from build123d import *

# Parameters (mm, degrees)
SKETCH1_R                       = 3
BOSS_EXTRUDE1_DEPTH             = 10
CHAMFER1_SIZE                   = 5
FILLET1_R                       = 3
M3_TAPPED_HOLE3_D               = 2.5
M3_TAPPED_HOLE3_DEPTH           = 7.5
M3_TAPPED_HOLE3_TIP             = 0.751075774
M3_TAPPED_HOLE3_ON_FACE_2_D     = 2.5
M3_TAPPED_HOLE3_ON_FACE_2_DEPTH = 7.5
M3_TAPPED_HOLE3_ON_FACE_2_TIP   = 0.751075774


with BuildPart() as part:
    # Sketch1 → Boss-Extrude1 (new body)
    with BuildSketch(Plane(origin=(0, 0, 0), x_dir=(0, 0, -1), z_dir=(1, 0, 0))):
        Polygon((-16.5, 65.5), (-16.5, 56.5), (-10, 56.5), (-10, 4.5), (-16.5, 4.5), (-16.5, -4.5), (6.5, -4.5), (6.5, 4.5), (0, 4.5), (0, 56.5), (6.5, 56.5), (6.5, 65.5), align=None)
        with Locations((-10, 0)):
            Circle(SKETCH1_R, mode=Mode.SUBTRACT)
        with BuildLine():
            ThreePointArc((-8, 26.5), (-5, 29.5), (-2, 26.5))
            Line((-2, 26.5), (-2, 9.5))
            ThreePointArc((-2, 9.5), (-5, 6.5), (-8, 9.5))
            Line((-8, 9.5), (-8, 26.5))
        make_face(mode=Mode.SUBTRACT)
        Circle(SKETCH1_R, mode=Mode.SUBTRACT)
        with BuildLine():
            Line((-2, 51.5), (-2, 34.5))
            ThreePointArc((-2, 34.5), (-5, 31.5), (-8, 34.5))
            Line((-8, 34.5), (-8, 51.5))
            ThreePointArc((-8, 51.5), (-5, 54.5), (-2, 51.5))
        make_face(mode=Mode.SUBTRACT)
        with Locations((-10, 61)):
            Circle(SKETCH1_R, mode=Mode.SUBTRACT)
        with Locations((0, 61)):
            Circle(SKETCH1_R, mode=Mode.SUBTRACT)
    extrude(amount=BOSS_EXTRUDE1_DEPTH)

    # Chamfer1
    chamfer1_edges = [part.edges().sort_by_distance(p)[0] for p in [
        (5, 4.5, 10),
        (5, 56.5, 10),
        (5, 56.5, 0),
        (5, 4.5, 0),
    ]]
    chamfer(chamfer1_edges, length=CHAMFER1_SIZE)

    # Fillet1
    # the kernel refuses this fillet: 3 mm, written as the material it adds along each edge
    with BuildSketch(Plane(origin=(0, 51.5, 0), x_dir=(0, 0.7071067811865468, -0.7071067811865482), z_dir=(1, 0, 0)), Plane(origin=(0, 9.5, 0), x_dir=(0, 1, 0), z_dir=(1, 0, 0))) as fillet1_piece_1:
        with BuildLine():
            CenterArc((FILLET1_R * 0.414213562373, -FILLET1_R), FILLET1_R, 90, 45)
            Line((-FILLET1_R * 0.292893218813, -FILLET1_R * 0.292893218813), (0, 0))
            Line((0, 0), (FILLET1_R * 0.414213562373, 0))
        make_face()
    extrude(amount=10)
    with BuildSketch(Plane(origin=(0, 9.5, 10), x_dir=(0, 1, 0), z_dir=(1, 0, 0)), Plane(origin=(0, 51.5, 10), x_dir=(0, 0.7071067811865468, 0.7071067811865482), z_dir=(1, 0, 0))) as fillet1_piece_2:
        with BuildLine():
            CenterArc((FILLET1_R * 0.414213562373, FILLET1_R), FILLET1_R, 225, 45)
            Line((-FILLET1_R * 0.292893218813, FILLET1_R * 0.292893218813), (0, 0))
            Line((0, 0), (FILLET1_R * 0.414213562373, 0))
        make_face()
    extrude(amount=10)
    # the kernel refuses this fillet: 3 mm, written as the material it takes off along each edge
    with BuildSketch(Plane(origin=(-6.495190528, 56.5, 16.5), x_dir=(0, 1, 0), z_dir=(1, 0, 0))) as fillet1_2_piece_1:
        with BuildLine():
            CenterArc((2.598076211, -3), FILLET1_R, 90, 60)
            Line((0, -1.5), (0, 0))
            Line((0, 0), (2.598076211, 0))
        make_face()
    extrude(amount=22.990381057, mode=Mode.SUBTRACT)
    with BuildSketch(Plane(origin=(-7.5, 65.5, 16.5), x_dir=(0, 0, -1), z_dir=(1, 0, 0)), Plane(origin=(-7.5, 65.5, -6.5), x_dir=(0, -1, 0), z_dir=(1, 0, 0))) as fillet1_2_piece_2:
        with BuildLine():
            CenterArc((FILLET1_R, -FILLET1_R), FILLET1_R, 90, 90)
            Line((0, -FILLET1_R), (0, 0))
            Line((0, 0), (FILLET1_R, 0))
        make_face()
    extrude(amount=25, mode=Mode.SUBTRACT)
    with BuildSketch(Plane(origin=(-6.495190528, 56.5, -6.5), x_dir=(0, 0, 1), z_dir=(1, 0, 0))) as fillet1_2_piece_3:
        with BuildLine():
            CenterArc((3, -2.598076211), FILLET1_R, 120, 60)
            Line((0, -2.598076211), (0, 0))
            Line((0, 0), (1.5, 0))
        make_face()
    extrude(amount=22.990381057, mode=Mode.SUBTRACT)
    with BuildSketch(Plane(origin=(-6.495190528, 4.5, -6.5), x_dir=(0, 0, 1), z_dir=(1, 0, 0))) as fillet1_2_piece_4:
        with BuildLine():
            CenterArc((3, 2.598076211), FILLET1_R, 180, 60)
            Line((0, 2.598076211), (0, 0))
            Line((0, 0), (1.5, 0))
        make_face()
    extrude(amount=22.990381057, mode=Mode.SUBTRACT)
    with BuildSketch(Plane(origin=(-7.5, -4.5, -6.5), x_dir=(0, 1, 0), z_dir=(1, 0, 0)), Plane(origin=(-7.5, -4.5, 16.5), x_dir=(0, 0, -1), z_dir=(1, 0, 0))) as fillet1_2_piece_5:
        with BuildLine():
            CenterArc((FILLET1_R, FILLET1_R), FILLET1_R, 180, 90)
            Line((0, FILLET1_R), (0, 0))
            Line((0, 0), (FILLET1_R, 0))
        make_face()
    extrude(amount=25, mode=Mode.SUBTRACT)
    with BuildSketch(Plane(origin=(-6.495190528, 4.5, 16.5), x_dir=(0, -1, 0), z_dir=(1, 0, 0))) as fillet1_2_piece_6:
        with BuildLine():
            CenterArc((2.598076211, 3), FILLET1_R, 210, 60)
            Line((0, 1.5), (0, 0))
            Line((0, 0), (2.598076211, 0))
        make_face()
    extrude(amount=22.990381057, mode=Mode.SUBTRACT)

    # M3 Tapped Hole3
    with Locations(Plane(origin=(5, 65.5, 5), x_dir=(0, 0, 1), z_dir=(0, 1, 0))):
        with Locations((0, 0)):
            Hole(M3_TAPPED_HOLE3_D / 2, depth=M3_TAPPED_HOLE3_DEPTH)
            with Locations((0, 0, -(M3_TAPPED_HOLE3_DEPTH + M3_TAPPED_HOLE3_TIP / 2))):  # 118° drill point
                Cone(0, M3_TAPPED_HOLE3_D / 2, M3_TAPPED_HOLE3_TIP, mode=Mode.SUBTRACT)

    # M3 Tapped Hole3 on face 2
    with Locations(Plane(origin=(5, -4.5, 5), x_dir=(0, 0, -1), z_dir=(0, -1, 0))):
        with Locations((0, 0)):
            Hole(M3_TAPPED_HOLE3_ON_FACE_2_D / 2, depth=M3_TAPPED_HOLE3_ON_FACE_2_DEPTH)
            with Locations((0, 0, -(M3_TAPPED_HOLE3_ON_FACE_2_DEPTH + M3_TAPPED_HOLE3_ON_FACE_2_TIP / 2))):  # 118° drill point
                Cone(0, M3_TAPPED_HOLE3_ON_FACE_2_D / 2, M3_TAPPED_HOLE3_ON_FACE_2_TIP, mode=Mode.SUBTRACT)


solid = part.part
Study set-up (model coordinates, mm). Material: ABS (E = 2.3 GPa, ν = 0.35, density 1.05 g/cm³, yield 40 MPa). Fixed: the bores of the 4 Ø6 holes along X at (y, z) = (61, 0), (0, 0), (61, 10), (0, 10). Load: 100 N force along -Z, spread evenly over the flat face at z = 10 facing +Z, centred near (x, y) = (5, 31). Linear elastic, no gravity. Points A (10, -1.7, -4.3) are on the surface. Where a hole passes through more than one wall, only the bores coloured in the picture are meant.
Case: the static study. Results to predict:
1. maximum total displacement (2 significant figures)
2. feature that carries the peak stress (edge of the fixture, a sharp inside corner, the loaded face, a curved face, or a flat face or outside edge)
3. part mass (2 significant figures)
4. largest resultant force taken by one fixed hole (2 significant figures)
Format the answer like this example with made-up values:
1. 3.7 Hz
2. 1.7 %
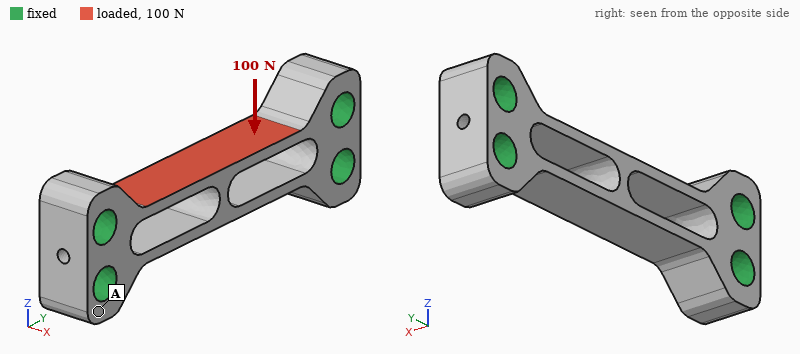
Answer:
1. 0.65 mm
2. a curved face
3. 6.2 g
4. 58 N
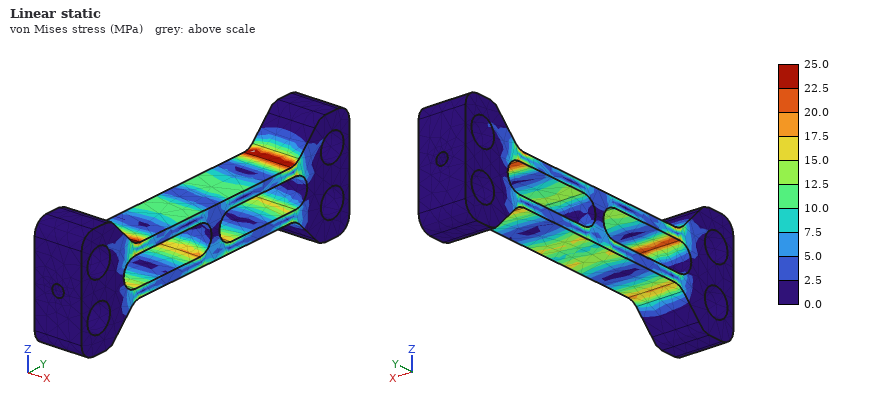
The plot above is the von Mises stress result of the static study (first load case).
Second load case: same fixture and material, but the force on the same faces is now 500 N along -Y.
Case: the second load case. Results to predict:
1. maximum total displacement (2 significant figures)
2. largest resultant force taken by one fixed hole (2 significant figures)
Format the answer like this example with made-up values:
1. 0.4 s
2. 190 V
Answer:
1. 88 µm
2. 210 N
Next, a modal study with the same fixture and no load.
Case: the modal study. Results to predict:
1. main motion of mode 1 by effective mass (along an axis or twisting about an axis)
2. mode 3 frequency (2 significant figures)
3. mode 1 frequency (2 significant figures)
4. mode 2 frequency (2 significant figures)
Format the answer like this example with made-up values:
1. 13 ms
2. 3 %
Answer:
1. along Z
2. 4600 Hz
3. 1500 Hz
4. 4500 Hz
